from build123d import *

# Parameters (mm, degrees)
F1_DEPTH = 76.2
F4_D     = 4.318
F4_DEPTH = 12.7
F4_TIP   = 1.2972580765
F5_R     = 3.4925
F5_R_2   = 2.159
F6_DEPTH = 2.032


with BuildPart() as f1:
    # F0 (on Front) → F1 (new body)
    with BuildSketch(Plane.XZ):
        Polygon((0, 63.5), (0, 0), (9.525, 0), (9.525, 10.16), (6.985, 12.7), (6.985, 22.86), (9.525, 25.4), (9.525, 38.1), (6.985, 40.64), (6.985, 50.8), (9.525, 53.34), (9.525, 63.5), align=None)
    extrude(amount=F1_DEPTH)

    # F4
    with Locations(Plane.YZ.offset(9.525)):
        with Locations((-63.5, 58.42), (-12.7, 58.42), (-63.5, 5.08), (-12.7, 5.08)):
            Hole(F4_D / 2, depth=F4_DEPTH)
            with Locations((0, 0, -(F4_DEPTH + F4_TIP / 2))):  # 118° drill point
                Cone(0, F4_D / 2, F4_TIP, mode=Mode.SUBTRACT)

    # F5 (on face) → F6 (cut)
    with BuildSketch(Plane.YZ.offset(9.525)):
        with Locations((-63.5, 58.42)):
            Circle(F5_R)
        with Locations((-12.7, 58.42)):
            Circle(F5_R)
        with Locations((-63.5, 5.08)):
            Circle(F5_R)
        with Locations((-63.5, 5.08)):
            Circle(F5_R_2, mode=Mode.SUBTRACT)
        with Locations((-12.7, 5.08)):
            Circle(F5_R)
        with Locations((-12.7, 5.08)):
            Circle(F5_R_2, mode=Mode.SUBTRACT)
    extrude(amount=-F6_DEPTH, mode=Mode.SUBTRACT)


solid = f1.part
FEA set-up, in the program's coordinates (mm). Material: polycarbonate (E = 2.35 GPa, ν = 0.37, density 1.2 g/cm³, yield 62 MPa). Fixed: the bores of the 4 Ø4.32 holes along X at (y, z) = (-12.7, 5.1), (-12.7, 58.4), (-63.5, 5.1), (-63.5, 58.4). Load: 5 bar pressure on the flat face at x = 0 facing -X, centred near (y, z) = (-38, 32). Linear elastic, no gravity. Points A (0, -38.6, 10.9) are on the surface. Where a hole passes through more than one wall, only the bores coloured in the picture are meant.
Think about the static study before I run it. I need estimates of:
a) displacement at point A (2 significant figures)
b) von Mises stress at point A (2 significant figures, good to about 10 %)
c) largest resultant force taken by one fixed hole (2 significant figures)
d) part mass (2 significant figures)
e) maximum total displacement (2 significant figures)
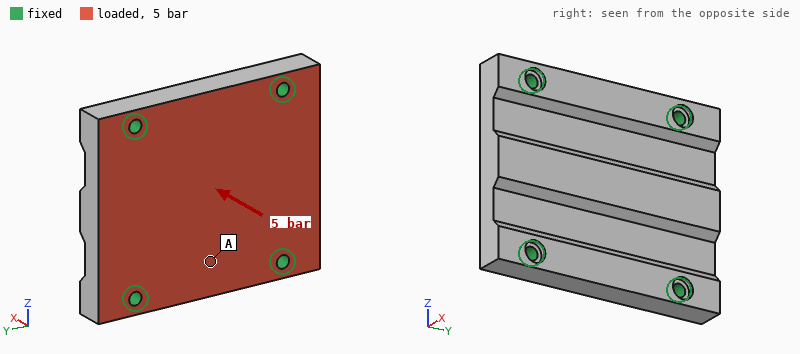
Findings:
0.18 mm
4.9 MPa
600 N
49 g
0.27 mm
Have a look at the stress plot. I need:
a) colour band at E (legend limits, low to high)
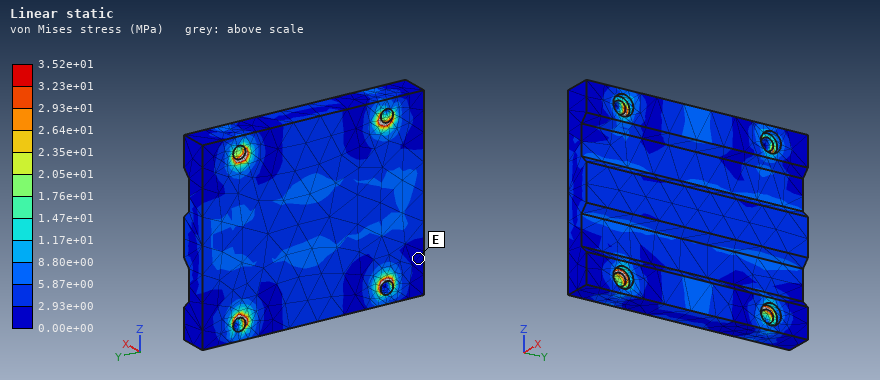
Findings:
0.00e+00 to 2.93e+00 MPa
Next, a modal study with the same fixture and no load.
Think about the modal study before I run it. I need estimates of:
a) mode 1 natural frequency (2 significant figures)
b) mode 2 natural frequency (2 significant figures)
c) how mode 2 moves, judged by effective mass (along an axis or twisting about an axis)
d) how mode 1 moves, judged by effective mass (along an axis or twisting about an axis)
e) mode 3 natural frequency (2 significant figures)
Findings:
2500 Hz
3300 Hz
twisting about Z
along X
3600 Hz
